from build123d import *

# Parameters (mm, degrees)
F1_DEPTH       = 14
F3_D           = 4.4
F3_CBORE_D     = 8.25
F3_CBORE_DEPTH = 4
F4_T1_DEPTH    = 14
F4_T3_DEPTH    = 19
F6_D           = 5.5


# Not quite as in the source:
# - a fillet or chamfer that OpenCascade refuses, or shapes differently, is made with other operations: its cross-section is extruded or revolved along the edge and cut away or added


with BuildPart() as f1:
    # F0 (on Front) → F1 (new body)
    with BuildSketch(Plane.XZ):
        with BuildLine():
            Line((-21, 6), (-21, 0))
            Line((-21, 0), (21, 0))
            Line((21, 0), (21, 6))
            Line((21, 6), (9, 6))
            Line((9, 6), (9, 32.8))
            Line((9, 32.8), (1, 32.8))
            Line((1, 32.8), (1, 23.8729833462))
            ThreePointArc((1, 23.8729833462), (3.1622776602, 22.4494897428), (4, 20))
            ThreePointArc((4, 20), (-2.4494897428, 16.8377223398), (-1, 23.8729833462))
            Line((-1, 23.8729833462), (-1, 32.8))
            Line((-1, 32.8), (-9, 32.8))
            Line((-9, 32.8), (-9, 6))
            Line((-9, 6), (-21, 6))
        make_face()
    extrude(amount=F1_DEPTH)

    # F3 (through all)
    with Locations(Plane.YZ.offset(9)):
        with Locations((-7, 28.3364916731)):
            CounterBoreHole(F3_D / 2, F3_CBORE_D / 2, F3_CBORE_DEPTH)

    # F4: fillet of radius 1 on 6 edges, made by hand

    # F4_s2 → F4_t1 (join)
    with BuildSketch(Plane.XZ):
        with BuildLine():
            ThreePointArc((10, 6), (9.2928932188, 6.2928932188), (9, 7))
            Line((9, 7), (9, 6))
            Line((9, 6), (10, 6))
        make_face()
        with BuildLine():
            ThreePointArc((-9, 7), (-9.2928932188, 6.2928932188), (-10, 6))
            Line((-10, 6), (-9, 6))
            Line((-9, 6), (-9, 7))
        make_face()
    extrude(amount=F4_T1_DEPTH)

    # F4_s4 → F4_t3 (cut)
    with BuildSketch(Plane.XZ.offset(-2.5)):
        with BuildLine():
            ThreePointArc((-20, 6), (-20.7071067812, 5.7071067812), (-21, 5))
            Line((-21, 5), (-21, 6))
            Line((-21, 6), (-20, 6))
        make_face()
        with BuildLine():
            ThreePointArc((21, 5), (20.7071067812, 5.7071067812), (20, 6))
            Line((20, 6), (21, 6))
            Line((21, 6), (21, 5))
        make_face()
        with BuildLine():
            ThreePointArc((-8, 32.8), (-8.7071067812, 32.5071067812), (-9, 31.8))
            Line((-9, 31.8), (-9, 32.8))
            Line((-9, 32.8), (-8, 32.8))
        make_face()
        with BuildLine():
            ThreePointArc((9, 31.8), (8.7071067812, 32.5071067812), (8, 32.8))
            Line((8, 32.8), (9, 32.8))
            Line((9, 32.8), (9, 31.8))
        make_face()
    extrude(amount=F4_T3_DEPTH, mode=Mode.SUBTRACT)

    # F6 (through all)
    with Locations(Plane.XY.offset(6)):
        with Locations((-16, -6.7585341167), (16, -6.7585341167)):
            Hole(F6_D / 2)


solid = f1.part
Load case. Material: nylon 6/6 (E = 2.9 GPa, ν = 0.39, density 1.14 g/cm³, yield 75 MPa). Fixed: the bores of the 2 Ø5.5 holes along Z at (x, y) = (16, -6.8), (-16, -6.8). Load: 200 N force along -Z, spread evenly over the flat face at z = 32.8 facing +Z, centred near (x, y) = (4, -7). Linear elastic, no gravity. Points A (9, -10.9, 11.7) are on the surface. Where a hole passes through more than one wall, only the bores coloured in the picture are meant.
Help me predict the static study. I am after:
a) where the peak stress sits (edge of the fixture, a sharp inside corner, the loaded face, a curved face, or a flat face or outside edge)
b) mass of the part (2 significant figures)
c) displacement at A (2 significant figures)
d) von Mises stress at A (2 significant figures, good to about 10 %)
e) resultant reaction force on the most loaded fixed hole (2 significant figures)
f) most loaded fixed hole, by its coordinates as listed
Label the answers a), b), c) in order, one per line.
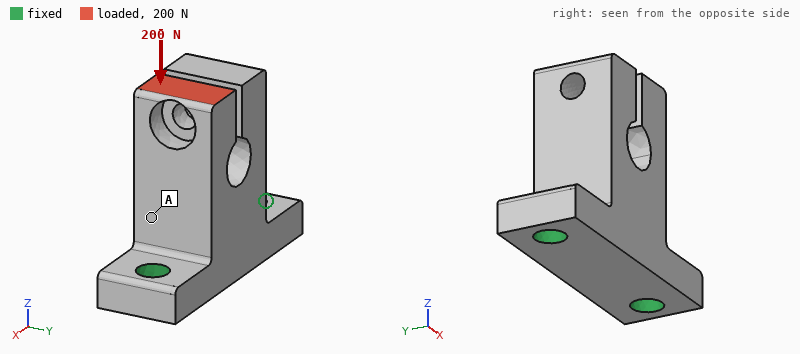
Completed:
a) the loaded face
b) 9.9 g
c) 0.025 mm
d) 1.9 MPa
e) 140 N
f) (16, -6.8)
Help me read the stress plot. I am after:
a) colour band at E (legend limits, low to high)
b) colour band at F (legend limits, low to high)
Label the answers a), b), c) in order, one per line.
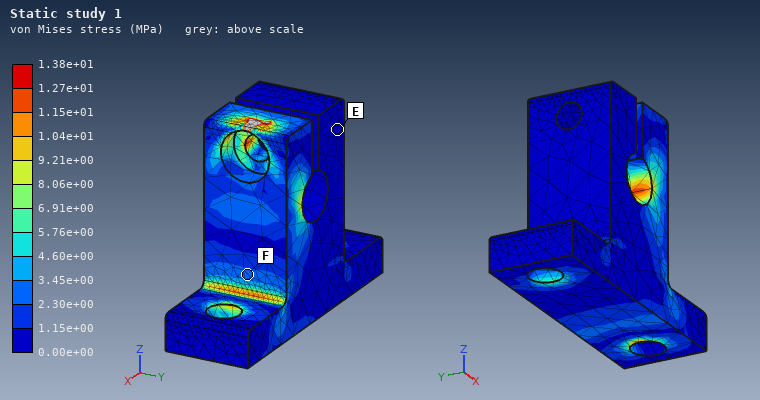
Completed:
a) 0.00e+00 to 1.15e+00 MPa
b) 2.30e+00 to 3.45e+00 MPa
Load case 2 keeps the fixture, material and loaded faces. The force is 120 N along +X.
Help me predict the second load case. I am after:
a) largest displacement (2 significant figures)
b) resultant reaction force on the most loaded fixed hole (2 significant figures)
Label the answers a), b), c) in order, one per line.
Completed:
a) 0.62 mm
b) 170 N
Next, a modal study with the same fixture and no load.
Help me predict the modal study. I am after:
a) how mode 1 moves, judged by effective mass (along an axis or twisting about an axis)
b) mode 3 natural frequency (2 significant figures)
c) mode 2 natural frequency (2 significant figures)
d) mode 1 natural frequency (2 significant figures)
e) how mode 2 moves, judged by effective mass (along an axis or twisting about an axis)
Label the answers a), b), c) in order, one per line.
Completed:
a) along Y
b) 3500 Hz
c) 2800 Hz
d) 1700 Hz
e) along X
